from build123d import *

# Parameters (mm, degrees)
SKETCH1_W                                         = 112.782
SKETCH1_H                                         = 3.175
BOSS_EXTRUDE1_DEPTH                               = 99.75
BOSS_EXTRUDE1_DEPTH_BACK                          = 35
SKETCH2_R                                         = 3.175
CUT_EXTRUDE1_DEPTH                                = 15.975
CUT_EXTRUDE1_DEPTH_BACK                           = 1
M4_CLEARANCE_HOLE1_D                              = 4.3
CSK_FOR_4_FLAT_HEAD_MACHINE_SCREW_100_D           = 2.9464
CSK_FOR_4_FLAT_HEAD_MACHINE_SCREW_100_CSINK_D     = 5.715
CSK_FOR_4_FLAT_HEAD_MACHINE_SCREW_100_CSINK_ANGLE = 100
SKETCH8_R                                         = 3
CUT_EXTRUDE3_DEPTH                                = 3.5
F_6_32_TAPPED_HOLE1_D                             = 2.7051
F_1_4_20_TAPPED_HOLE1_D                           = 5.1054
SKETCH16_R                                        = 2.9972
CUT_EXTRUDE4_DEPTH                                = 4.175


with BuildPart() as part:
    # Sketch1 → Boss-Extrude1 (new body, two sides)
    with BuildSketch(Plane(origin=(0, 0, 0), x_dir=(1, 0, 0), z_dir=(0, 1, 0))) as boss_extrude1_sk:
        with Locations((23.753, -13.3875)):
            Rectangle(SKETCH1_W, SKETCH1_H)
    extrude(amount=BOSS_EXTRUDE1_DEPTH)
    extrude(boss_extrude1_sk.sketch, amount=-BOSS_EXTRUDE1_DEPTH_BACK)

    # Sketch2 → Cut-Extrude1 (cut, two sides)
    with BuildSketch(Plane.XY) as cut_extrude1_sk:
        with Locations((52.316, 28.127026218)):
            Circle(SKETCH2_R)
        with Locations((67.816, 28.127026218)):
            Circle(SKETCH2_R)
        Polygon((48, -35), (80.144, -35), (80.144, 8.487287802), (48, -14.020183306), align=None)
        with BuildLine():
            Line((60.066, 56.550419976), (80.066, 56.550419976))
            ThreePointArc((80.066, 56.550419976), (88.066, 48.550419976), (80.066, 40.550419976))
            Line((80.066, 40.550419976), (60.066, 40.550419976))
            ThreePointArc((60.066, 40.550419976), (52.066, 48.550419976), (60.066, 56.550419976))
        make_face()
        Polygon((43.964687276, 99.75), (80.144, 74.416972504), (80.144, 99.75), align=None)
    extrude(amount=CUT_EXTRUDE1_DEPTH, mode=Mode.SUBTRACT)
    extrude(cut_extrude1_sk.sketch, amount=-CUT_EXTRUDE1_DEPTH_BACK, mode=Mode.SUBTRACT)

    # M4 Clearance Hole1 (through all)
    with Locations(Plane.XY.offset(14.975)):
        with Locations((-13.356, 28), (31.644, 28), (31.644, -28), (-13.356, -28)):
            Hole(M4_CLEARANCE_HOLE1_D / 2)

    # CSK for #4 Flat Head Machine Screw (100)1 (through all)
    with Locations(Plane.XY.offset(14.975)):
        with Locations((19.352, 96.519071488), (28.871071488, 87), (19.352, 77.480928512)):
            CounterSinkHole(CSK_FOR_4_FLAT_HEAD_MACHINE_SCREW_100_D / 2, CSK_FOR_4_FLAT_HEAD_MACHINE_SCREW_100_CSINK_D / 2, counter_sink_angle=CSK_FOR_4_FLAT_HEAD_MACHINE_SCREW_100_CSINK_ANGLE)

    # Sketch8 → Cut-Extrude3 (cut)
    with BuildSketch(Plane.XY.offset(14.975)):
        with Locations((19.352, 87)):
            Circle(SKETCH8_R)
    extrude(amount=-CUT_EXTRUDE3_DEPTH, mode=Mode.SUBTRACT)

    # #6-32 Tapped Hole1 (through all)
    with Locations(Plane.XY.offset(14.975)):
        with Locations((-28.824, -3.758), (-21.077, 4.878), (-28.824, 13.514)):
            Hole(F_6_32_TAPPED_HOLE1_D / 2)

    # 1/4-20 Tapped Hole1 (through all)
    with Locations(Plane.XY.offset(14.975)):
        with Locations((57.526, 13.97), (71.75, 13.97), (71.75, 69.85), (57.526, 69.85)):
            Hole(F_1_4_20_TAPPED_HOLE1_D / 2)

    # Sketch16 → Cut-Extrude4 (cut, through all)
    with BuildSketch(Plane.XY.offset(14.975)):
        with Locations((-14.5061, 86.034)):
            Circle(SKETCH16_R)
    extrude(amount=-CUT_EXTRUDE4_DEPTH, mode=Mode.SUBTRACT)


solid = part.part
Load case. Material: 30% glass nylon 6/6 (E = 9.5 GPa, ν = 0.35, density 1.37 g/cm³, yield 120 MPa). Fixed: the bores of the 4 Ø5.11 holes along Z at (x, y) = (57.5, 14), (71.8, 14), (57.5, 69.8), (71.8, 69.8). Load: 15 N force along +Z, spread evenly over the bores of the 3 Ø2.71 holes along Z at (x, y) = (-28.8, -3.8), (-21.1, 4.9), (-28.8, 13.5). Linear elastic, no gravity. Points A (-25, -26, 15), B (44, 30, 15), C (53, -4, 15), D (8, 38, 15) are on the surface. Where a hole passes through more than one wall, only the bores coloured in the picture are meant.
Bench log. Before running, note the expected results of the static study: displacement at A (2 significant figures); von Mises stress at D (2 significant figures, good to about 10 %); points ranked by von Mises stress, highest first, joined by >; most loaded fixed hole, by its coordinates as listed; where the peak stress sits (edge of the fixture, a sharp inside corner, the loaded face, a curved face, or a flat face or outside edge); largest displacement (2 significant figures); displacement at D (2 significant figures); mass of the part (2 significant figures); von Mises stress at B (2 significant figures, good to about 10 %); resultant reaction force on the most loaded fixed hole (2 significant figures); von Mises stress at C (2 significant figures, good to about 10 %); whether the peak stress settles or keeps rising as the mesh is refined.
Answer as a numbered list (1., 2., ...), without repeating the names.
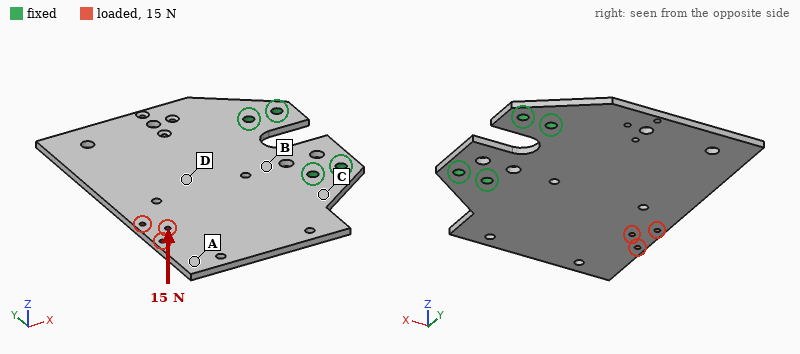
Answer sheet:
1. 1.5 mm
2. 3.1 MPa
3. C > B > D > A
4. (57.5, 14)
5. edge of the fixture
6. 1.7 mm
7. 0.51 mm
8. 56 g
9. 5.0 MPa
10. 40 N
11. 8.6 MPa
12. keeps rising
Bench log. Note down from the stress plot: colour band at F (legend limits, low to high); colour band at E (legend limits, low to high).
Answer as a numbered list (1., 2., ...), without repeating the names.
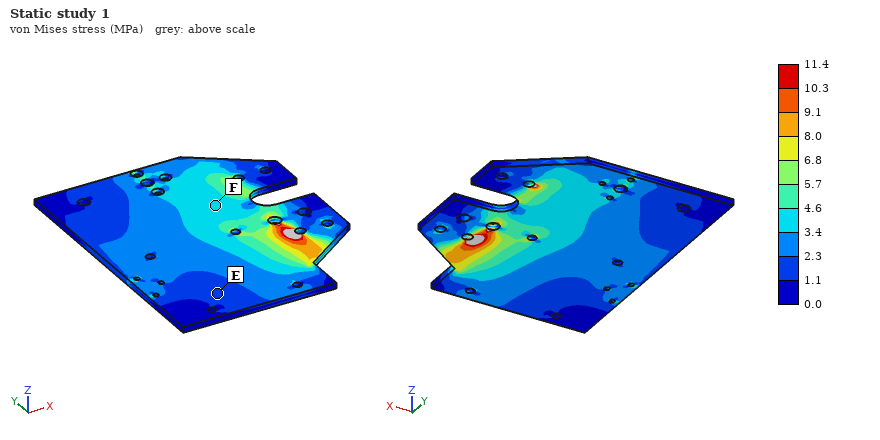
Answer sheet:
1. 3.4 to 4.6 MPa
2. 1.1 to 2.3 MPa
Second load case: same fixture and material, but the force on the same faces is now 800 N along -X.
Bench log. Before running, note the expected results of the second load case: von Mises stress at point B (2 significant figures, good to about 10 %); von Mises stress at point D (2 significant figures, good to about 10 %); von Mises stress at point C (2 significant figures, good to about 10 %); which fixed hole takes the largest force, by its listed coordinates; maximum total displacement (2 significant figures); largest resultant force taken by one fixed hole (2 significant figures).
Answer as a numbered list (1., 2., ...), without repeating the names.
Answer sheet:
1. 3.2 MPa
2. 1.9 MPa
3. 5.6 MPa
4. (57.5, 14)
5. 97 µm
6. 620 N
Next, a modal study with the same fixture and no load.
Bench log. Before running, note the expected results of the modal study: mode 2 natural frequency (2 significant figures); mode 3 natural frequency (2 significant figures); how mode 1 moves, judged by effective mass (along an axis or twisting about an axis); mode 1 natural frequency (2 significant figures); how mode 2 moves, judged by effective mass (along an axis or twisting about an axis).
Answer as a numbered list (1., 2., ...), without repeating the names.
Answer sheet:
1. 250 Hz
2. 560 Hz
3. along Z
4. 140 Hz
5. twisting about X
